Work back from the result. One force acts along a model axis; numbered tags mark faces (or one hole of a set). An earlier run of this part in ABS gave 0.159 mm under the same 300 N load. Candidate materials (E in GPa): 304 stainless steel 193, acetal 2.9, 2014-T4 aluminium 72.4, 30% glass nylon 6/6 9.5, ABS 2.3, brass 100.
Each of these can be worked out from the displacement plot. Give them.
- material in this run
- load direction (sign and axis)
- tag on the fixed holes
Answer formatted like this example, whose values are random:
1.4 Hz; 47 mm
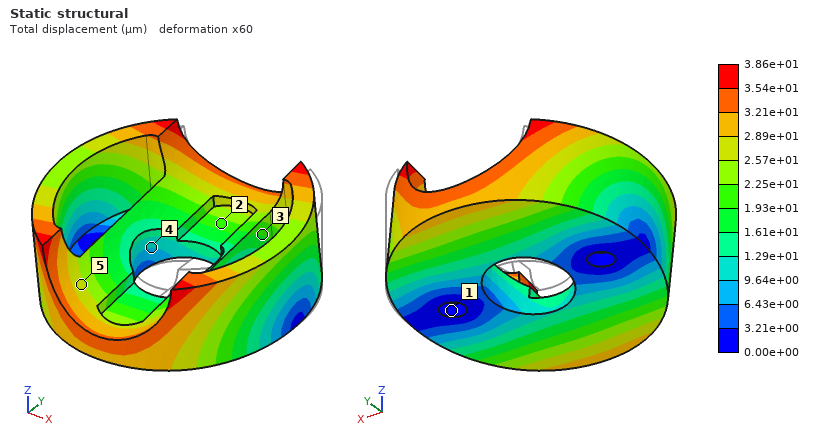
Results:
30% glass nylon 6/6; -Y; 1
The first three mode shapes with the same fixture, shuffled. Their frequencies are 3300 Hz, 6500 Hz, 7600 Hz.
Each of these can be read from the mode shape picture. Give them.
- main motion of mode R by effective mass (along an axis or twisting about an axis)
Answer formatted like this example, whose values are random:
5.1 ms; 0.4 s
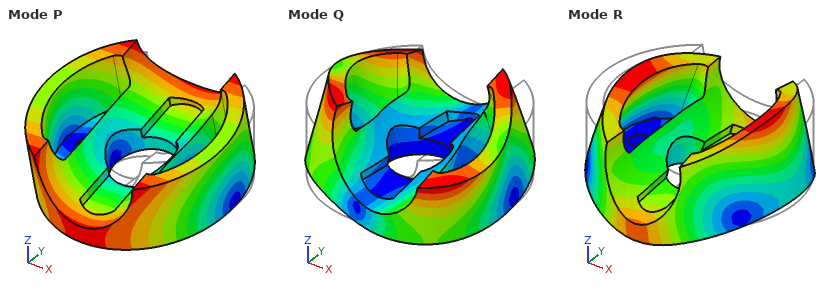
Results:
along Z
